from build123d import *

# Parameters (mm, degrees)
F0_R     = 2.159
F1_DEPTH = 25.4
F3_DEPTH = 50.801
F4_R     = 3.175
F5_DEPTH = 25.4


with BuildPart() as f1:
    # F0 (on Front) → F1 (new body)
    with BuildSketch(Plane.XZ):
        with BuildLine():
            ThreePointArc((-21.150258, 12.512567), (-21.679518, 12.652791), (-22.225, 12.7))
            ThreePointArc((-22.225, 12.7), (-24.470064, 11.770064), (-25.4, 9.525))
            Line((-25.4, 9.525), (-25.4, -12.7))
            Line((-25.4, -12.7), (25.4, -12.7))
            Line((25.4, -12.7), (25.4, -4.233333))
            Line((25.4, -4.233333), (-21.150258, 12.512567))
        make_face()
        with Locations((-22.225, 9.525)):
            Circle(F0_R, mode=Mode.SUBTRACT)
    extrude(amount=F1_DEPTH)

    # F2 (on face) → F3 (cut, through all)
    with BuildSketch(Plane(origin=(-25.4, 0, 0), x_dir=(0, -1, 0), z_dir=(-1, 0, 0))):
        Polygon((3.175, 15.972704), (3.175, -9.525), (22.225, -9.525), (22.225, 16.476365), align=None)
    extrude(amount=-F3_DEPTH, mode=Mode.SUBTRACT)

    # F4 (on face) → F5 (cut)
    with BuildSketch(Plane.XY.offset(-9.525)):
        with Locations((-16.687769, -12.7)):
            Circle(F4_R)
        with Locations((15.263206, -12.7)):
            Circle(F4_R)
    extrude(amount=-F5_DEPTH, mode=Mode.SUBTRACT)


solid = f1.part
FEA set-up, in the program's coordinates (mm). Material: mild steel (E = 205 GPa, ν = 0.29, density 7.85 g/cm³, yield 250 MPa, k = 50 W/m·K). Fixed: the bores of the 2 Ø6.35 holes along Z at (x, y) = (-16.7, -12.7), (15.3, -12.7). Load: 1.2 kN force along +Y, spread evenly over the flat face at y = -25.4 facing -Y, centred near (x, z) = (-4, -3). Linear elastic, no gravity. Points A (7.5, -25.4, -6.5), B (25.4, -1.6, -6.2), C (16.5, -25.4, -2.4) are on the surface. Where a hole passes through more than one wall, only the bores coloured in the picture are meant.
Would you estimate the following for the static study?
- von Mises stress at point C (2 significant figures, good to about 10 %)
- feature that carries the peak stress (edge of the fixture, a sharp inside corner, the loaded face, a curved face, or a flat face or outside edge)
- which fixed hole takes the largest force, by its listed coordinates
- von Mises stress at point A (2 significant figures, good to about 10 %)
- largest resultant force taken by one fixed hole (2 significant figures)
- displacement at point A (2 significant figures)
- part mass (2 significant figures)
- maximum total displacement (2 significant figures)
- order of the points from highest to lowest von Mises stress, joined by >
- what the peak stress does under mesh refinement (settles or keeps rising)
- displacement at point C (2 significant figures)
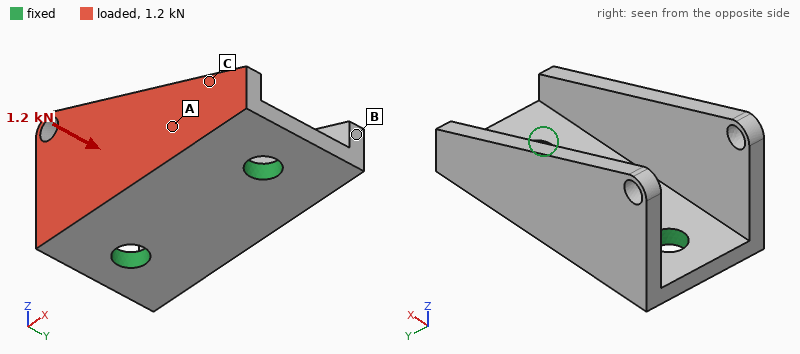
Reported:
35 MPa
edge of the fixture
(-16.7, -12.7)
60 MPa
720 N
0.025 mm
66 g
0.14 mm
A > C > B
keeps rising
0.029 mm
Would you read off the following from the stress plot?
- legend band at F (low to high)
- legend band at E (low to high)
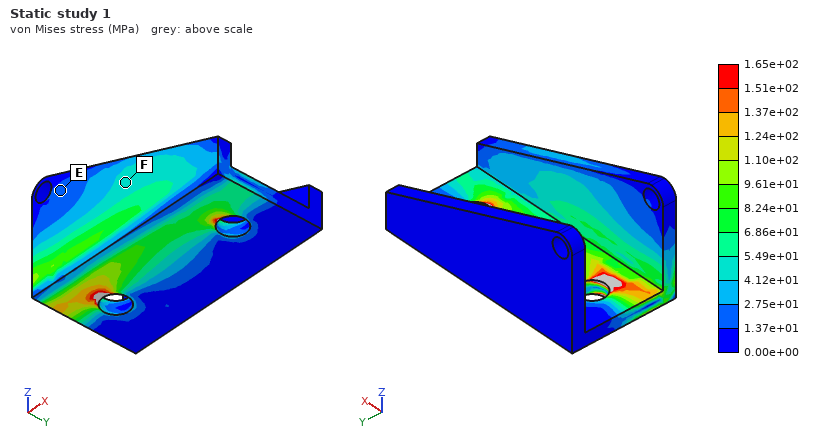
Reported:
4.12e+01 to 5.49e+01 MPa
1.37e+01 to 2.75e+01 MPa
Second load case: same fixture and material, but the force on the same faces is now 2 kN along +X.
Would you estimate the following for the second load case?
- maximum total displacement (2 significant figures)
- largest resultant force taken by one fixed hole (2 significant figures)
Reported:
20 µm
1.3 kN
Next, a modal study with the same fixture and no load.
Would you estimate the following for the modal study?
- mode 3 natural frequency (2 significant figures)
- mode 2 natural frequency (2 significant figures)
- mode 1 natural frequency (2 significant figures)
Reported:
8700 Hz
4300 Hz
4200 Hz
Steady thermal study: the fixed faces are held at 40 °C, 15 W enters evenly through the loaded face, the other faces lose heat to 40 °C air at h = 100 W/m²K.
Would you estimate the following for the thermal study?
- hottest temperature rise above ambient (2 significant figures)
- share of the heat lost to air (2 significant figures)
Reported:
32 K
28 %
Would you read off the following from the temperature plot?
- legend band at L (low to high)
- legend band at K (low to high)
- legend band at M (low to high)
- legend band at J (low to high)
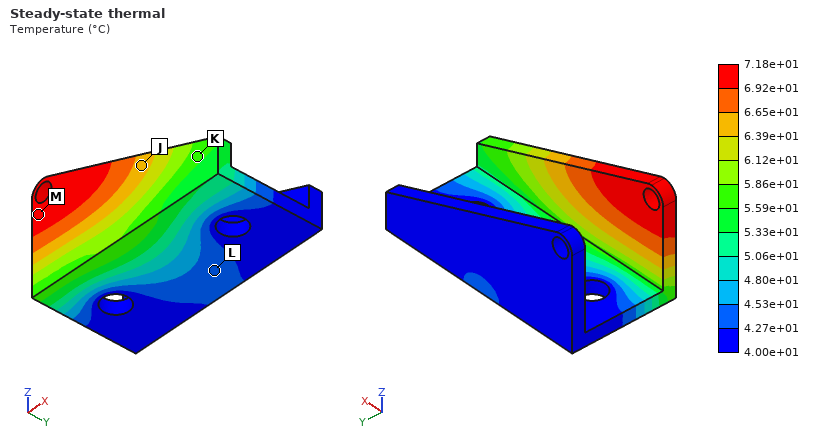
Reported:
4.27e+01 to 4.53e+01 °C
5.59e+01 to 5.86e+01 °C
6.92e+01 to 7.18e+01 °C
6.39e+01 to 6.65e+01 °C
